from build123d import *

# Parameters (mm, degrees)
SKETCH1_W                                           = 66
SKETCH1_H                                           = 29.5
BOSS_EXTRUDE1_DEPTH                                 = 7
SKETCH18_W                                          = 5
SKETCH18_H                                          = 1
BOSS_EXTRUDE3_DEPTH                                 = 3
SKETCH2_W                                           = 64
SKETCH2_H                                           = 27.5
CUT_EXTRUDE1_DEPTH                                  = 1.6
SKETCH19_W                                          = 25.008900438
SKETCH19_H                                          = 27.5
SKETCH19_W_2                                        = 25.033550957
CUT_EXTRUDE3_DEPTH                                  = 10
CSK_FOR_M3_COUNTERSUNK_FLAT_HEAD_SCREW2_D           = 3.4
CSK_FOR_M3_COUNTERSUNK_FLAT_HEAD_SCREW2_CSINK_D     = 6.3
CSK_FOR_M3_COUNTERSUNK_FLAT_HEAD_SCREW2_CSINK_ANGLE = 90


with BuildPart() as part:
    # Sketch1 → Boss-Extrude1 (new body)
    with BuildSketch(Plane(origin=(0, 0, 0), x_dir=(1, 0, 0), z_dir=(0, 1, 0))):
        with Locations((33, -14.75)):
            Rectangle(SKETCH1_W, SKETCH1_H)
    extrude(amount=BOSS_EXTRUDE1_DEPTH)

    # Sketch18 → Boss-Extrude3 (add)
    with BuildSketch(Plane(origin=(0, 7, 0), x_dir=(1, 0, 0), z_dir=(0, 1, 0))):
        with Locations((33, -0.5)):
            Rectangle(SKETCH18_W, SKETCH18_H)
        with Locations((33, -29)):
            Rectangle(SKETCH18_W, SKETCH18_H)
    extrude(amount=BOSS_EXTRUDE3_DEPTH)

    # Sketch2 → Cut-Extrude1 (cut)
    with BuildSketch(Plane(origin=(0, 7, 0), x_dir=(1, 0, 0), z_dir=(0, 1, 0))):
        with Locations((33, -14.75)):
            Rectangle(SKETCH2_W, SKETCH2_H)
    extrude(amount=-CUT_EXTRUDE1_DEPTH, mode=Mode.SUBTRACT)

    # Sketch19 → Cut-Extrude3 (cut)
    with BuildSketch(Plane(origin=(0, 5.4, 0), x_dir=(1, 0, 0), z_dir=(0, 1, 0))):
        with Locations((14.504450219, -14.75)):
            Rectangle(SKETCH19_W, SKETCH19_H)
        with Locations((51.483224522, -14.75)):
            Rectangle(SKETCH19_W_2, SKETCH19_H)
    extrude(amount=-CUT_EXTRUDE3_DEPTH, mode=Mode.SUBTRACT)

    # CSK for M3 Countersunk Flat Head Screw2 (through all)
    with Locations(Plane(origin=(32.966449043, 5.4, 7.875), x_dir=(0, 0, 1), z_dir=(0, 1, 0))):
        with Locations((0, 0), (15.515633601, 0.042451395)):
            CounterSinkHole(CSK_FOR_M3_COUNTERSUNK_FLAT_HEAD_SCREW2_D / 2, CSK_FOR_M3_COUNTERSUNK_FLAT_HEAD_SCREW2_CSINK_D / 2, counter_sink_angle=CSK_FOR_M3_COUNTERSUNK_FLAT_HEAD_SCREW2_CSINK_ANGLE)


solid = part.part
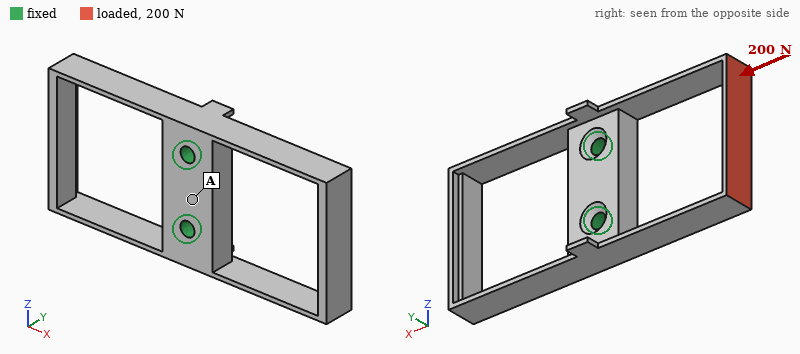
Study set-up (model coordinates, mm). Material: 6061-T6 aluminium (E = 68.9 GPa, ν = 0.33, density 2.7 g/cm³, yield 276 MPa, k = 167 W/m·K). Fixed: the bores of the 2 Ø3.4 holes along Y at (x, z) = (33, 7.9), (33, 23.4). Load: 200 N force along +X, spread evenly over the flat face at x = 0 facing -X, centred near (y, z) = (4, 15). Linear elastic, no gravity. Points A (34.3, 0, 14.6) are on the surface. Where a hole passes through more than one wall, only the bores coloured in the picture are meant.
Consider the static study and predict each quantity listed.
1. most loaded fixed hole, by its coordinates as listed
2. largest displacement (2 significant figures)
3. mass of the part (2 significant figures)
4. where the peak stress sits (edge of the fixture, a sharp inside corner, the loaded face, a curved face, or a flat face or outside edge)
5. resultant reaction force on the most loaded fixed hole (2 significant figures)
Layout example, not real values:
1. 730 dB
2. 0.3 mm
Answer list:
1. (33, 7.9)
2. 0.19 mm
3. 8.9 g
4. a flat face or outside edge
5. 110 N
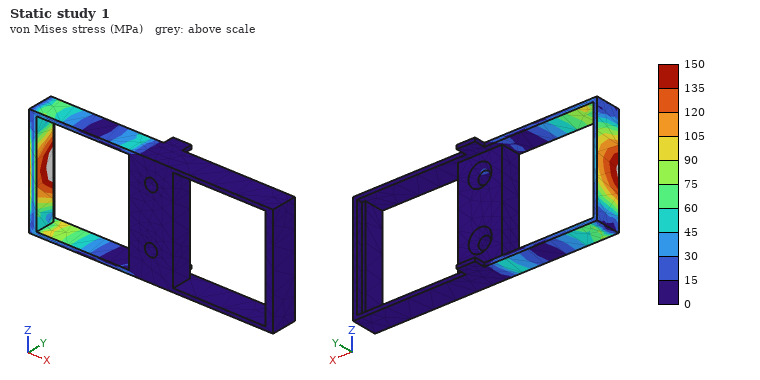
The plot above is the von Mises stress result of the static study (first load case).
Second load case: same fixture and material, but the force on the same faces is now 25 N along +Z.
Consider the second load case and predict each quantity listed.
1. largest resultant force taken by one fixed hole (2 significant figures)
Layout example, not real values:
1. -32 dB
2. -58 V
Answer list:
1. 40 N
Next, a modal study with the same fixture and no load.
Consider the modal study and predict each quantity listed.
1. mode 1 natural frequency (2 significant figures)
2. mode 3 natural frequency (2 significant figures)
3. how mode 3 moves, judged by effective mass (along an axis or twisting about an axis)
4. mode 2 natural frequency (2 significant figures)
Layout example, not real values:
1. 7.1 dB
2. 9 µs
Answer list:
1. 1000 Hz
2. 2700 Hz
3. twisting about Z
4. 1000 Hz
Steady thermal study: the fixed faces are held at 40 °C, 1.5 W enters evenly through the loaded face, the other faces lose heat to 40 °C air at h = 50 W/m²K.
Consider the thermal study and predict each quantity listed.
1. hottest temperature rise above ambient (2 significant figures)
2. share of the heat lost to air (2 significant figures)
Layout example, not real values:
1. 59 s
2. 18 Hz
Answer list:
1. 15 K
2. 35 %
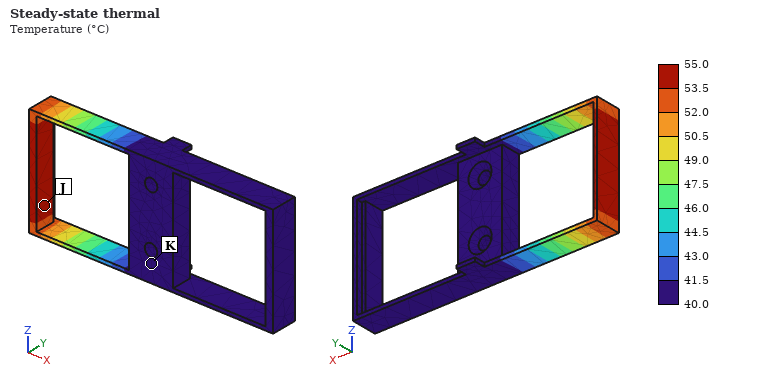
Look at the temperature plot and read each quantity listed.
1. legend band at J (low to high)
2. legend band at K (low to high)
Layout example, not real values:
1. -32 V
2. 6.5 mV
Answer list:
1. 53.5 to 55.0 °C
2. 40.0 to 41.5 °C
